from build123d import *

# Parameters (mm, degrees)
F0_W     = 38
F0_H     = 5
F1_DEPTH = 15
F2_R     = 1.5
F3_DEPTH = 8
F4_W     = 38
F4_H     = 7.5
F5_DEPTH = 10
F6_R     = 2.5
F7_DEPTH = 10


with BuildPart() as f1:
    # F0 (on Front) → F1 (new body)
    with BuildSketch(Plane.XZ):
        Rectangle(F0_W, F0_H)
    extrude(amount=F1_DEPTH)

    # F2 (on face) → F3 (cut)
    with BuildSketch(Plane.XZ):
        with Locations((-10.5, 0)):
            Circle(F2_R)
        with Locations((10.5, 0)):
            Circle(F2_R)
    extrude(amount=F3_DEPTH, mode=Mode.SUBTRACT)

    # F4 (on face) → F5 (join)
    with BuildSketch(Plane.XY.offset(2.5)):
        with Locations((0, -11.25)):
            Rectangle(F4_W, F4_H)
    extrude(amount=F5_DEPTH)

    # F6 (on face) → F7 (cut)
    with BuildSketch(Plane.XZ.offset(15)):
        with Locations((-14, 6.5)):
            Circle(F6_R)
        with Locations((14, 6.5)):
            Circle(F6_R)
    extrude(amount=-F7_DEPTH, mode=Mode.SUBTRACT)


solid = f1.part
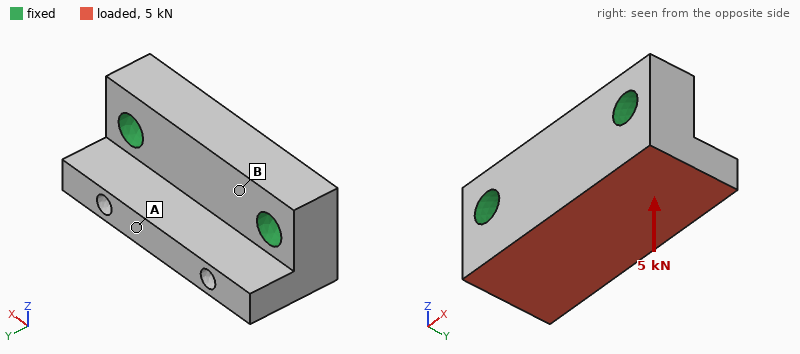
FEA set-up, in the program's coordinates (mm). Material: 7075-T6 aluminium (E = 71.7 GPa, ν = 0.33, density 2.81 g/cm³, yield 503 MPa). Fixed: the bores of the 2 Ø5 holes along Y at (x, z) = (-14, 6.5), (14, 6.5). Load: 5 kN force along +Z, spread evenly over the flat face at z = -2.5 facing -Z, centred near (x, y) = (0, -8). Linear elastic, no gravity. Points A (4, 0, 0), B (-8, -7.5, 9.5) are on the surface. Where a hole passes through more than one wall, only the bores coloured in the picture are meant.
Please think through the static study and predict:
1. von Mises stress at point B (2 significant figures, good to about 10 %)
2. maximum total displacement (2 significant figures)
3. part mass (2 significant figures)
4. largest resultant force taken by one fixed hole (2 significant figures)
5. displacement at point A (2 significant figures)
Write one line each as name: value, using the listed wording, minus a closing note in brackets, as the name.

von Mises stress at point B: 41 MPa
maximum total displacement: 38 µm
part mass: 15 g
largest resultant force taken by one fixed hole: 2.5 kN
displacement at point A: 35 µm
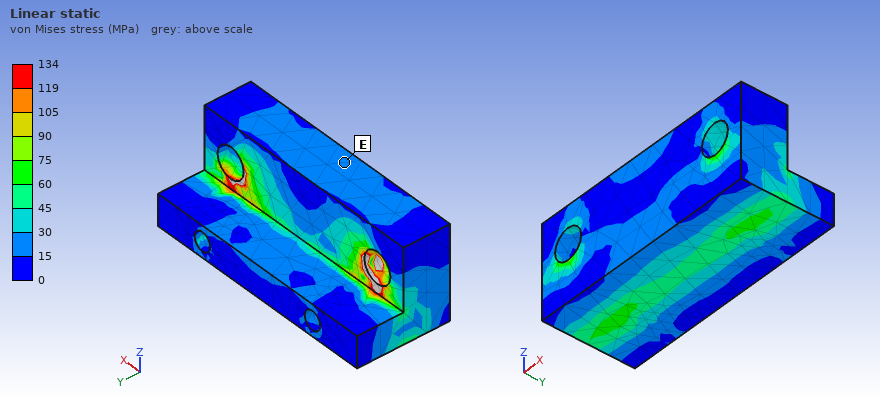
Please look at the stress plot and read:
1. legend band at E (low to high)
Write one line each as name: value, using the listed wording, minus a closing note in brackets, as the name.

legend band at E: 15 to 30 MPa
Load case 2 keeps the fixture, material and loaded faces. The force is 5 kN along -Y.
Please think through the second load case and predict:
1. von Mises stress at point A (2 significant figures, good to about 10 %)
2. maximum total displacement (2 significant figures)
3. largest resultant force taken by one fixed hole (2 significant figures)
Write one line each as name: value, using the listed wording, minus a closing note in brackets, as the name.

von Mises stress at point A: 29 MPa
maximum total displacement: 51 µm
largest resultant force taken by one fixed hole: 2.5 kN
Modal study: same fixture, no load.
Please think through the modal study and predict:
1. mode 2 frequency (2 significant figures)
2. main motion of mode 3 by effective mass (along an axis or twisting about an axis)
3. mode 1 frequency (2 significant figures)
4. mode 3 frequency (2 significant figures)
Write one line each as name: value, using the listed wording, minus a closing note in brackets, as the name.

mode 2 frequency: 34 kHz
main motion of mode 3 by effective mass: along Y
mode 1 frequency: 24 kHz
mode 3 frequency: 38 kHz
